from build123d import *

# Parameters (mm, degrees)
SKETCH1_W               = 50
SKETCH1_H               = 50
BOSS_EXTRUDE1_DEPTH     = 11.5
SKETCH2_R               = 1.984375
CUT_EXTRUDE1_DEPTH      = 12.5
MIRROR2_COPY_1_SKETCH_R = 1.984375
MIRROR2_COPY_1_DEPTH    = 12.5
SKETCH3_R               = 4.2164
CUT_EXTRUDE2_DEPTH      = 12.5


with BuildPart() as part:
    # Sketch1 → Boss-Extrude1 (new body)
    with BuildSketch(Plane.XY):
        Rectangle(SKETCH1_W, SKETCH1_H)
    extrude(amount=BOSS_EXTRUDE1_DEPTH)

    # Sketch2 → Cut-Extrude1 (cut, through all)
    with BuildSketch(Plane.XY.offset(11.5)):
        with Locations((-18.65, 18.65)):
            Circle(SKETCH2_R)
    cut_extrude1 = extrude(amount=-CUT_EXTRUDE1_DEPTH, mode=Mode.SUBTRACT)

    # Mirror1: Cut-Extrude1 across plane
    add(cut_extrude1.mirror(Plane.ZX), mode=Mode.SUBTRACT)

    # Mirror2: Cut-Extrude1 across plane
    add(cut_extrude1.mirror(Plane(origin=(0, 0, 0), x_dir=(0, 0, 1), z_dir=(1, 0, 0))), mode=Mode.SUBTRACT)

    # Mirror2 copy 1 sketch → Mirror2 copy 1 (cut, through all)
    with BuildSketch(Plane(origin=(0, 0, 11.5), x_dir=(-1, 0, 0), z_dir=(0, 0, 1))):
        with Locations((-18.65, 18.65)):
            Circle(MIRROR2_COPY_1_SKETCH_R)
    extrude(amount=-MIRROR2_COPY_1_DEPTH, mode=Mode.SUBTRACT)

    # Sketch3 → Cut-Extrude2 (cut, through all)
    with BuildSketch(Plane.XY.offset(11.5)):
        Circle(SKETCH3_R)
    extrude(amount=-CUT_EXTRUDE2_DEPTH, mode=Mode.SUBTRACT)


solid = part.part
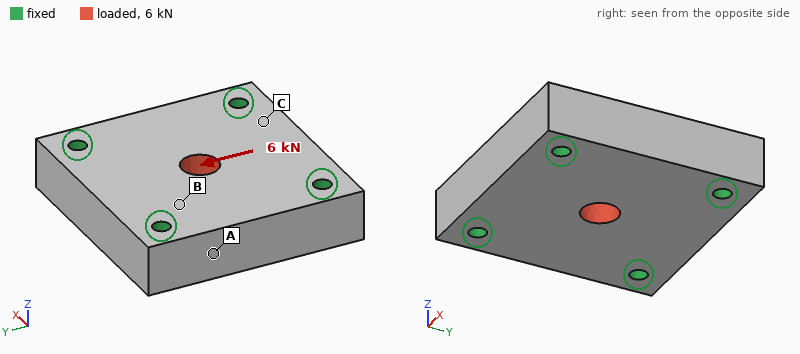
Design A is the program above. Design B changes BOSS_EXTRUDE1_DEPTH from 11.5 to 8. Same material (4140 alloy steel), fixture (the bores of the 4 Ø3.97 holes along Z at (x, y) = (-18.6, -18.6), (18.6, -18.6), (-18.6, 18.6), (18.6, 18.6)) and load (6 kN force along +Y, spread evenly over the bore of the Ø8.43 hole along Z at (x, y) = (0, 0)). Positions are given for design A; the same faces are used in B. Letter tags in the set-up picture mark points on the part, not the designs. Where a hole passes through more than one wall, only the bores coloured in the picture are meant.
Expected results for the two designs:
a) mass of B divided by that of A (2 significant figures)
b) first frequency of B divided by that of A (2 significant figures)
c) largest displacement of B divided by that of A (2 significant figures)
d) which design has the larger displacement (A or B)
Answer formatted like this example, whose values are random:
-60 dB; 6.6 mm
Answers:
0.70; 0.82; 1.4; B
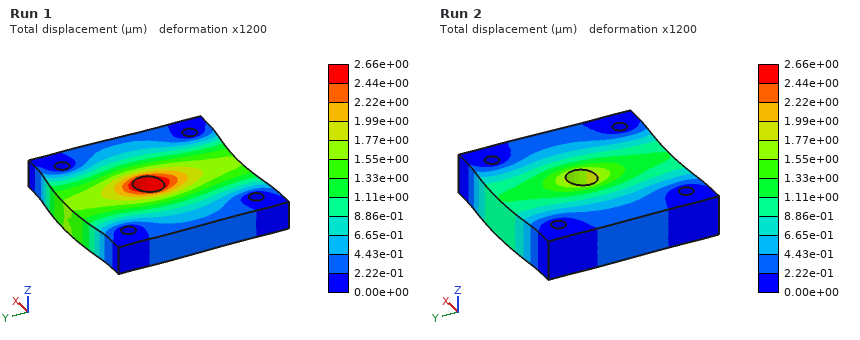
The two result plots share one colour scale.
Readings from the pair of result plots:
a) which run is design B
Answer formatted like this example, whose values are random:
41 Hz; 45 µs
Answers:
Run 1
